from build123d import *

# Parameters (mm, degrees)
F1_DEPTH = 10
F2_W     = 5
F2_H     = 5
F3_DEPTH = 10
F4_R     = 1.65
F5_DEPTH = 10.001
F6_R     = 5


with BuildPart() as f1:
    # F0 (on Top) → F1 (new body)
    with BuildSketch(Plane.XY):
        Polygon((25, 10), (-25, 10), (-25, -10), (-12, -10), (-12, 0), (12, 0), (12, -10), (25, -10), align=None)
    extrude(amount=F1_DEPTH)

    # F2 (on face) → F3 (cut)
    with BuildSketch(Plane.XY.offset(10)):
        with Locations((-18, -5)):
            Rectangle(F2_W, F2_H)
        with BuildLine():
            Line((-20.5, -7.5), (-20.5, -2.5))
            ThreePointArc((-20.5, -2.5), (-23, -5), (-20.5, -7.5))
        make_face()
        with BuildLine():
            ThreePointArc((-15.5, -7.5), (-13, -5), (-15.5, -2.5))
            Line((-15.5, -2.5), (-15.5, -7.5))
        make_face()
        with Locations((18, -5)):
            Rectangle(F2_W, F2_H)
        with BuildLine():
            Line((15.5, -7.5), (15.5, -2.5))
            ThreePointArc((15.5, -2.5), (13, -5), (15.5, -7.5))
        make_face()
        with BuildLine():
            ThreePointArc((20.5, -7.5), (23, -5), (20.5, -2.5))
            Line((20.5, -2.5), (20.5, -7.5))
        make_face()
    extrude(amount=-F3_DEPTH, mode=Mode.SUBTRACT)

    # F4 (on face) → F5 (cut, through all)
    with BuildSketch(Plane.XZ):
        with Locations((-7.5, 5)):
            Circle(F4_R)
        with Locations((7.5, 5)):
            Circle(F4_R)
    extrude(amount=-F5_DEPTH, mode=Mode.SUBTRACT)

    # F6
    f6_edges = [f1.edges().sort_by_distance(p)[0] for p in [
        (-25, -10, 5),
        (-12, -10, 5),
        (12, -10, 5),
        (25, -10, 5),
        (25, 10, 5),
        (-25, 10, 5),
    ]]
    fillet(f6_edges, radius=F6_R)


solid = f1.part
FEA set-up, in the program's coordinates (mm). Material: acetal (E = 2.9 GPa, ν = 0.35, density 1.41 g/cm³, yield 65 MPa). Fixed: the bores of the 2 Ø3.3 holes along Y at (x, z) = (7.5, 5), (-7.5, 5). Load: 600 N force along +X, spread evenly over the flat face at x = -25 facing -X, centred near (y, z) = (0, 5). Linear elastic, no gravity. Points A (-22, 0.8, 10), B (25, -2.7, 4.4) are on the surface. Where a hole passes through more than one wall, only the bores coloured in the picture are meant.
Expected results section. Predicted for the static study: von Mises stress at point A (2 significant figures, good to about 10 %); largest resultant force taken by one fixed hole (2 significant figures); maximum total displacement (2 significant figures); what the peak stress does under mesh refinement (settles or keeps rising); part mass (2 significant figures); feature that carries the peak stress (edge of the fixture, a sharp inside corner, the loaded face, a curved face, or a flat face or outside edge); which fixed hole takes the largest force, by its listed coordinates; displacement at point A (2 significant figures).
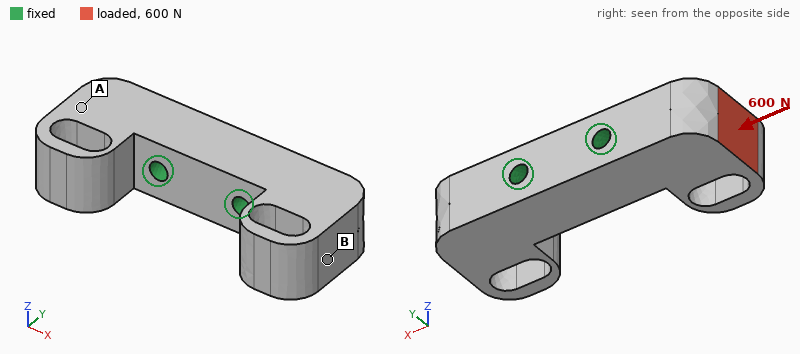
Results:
6.6 MPa
560 N
0.25 mm
keeps rising
8.8 g
edge of the fixture
(-7.5, 5)
0.13 mm
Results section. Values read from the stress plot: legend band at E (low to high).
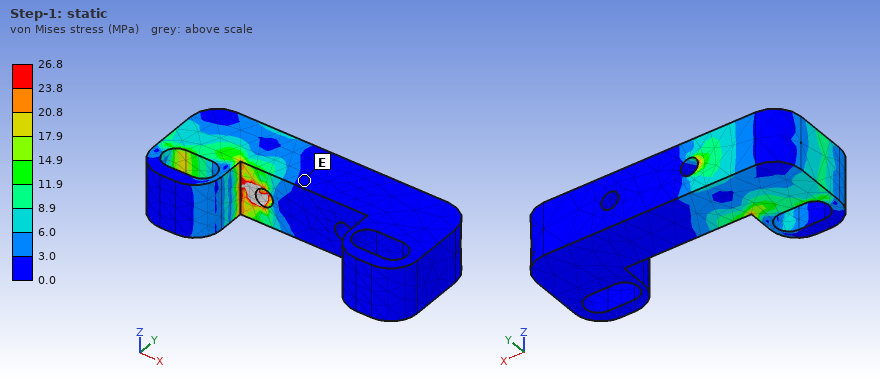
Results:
0.0 to 3.0 MPa
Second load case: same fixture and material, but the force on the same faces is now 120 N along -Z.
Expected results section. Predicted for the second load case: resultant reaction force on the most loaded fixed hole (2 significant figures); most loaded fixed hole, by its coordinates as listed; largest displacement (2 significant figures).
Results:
180 N
(-7.5, 5)
0.19 mm
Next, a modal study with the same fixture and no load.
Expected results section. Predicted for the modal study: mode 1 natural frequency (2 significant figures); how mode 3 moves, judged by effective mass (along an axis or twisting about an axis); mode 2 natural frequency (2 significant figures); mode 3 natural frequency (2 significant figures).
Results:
3900 Hz
along Y
3900 Hz
4300 Hz
